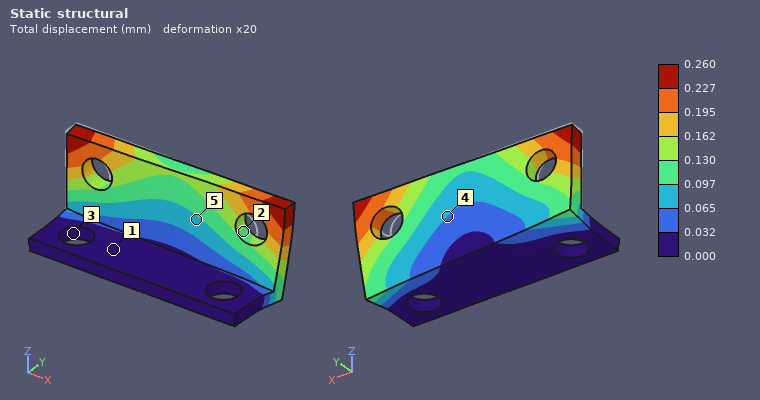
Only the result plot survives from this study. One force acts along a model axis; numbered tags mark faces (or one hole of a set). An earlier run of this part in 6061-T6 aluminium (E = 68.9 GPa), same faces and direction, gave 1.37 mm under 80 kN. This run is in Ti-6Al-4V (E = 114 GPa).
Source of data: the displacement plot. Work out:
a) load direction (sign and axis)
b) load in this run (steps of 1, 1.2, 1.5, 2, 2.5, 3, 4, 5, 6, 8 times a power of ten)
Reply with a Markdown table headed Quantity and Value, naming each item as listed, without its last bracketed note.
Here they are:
| Quantity | Value |
|---|---|
| load direction | +X |
| load in this run | 25 kN |
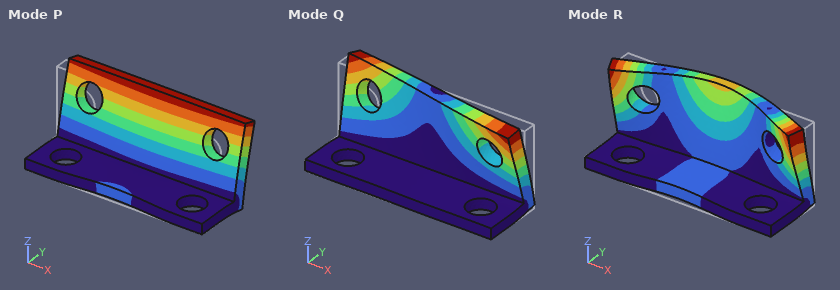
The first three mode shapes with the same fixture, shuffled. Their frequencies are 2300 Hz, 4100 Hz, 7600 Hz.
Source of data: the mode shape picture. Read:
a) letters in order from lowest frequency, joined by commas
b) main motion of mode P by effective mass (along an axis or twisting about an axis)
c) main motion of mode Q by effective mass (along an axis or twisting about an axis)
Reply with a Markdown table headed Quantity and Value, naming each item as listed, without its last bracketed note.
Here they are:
| Quantity | Value |
|---|---|
| letters in order from lowest frequency, joined by commas | P, Q, R |
| main motion of mode P by effective mass | along Y |
| main motion of mode Q by effective mass | twisting about Z |
